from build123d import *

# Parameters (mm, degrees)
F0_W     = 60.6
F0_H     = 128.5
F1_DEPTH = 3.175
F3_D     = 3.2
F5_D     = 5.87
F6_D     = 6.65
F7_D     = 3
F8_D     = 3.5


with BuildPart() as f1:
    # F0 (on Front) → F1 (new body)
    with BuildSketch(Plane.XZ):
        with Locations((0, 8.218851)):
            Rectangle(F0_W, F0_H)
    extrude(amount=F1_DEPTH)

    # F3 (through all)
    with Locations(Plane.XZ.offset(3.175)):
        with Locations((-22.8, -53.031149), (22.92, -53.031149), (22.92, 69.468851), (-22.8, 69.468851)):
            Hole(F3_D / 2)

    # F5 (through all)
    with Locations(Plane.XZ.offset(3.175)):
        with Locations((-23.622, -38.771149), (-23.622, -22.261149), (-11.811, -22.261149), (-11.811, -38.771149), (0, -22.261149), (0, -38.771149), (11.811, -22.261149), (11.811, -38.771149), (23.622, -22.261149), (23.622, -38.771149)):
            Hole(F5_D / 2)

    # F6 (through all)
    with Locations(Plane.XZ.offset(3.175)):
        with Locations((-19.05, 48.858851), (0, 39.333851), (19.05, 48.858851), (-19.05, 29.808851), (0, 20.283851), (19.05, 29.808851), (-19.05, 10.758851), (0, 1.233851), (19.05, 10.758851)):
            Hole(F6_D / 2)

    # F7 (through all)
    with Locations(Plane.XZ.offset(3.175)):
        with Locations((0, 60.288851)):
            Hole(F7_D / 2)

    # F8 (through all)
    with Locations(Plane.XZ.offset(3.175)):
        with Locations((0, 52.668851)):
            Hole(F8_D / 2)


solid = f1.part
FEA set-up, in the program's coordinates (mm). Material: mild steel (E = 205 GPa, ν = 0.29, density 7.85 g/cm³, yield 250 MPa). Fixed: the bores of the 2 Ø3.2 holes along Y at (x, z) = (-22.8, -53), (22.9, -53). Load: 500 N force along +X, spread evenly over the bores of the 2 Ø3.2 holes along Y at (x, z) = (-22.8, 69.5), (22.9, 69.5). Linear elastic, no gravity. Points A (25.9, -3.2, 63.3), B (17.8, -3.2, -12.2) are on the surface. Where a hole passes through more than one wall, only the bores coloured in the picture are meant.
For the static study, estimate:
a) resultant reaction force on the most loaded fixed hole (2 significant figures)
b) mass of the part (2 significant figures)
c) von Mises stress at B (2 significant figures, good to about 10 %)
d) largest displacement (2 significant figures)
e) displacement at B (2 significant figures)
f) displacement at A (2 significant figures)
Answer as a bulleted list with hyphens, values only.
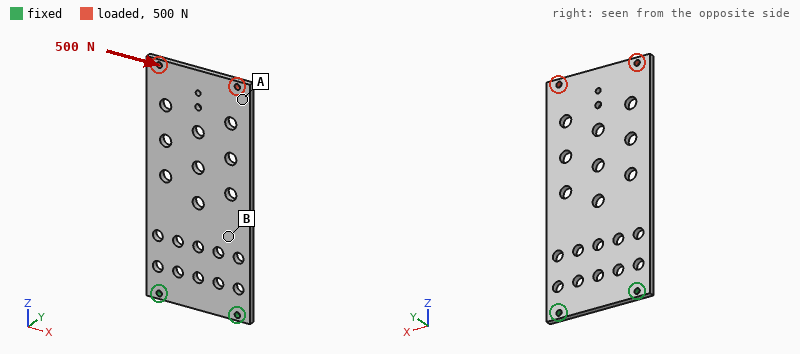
- 1.3 kN
- 180 g
- 14 MPa
- 47 µm
- 10 µm
- 42 µm
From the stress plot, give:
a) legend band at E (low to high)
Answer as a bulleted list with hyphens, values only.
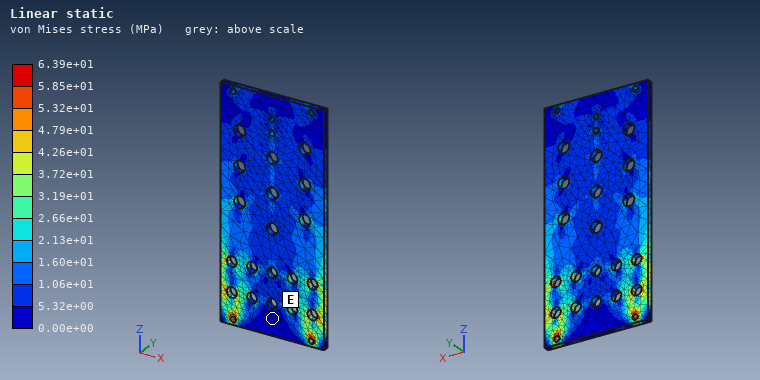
- 0.00e+00 to 5.32e+00 MPa
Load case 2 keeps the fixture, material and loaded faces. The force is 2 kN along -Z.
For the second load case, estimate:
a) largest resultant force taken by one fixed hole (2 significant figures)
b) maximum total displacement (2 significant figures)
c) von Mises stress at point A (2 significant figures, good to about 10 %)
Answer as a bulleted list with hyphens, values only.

- 1.0 kN
- 12 µm
- 25 MPa
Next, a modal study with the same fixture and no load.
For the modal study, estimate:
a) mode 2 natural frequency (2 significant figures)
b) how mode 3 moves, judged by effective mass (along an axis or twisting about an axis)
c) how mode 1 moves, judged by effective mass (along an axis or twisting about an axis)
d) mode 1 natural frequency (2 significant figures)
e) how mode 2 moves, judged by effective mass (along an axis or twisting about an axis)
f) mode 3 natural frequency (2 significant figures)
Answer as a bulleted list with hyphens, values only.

- 710 Hz
- along Y
- along Y
- 140 Hz
- twisting about Z
- 950 Hz
